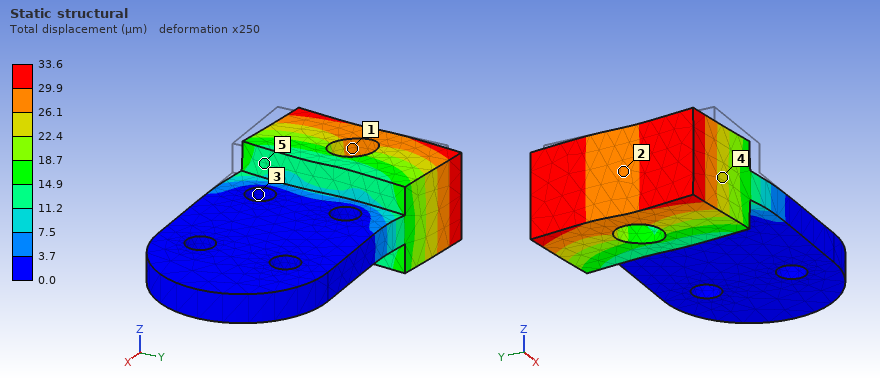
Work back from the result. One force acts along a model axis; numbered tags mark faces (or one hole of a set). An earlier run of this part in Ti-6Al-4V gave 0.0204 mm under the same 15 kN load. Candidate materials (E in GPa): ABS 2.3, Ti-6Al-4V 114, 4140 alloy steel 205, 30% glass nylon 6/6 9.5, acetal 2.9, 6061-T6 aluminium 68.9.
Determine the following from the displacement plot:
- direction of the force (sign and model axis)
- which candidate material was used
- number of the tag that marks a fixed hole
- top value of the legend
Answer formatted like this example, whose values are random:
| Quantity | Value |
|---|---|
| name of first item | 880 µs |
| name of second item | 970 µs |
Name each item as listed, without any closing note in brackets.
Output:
| Quantity | Value |
|---|---|
| direction of the force | +Y |
| which candidate material was used | 6061-T6 aluminium |
| number of the tag that marks a fixed hole | 3 |
| top value of the legend | 33.6 µm |
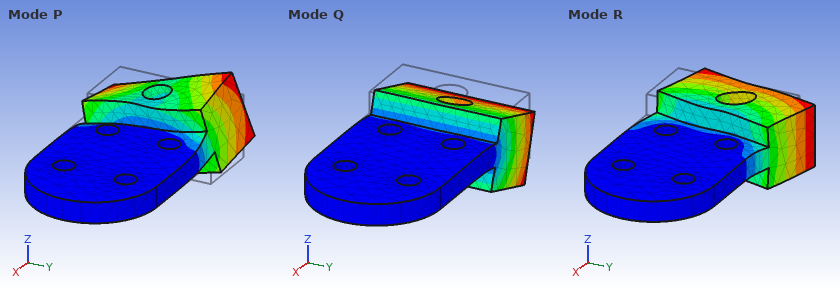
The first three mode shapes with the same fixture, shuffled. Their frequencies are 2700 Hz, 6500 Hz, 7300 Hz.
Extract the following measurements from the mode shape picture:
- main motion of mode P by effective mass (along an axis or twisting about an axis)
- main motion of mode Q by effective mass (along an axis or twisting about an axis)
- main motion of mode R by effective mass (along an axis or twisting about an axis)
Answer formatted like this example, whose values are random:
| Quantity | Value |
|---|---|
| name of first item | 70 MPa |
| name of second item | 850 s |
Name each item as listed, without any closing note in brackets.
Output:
| Quantity | Value |
|---|---|
| main motion of mode P by effective mass | twisting about X |
| main motion of mode Q by effective mass | along Z |
| main motion of mode R by effective mass | along Y |
